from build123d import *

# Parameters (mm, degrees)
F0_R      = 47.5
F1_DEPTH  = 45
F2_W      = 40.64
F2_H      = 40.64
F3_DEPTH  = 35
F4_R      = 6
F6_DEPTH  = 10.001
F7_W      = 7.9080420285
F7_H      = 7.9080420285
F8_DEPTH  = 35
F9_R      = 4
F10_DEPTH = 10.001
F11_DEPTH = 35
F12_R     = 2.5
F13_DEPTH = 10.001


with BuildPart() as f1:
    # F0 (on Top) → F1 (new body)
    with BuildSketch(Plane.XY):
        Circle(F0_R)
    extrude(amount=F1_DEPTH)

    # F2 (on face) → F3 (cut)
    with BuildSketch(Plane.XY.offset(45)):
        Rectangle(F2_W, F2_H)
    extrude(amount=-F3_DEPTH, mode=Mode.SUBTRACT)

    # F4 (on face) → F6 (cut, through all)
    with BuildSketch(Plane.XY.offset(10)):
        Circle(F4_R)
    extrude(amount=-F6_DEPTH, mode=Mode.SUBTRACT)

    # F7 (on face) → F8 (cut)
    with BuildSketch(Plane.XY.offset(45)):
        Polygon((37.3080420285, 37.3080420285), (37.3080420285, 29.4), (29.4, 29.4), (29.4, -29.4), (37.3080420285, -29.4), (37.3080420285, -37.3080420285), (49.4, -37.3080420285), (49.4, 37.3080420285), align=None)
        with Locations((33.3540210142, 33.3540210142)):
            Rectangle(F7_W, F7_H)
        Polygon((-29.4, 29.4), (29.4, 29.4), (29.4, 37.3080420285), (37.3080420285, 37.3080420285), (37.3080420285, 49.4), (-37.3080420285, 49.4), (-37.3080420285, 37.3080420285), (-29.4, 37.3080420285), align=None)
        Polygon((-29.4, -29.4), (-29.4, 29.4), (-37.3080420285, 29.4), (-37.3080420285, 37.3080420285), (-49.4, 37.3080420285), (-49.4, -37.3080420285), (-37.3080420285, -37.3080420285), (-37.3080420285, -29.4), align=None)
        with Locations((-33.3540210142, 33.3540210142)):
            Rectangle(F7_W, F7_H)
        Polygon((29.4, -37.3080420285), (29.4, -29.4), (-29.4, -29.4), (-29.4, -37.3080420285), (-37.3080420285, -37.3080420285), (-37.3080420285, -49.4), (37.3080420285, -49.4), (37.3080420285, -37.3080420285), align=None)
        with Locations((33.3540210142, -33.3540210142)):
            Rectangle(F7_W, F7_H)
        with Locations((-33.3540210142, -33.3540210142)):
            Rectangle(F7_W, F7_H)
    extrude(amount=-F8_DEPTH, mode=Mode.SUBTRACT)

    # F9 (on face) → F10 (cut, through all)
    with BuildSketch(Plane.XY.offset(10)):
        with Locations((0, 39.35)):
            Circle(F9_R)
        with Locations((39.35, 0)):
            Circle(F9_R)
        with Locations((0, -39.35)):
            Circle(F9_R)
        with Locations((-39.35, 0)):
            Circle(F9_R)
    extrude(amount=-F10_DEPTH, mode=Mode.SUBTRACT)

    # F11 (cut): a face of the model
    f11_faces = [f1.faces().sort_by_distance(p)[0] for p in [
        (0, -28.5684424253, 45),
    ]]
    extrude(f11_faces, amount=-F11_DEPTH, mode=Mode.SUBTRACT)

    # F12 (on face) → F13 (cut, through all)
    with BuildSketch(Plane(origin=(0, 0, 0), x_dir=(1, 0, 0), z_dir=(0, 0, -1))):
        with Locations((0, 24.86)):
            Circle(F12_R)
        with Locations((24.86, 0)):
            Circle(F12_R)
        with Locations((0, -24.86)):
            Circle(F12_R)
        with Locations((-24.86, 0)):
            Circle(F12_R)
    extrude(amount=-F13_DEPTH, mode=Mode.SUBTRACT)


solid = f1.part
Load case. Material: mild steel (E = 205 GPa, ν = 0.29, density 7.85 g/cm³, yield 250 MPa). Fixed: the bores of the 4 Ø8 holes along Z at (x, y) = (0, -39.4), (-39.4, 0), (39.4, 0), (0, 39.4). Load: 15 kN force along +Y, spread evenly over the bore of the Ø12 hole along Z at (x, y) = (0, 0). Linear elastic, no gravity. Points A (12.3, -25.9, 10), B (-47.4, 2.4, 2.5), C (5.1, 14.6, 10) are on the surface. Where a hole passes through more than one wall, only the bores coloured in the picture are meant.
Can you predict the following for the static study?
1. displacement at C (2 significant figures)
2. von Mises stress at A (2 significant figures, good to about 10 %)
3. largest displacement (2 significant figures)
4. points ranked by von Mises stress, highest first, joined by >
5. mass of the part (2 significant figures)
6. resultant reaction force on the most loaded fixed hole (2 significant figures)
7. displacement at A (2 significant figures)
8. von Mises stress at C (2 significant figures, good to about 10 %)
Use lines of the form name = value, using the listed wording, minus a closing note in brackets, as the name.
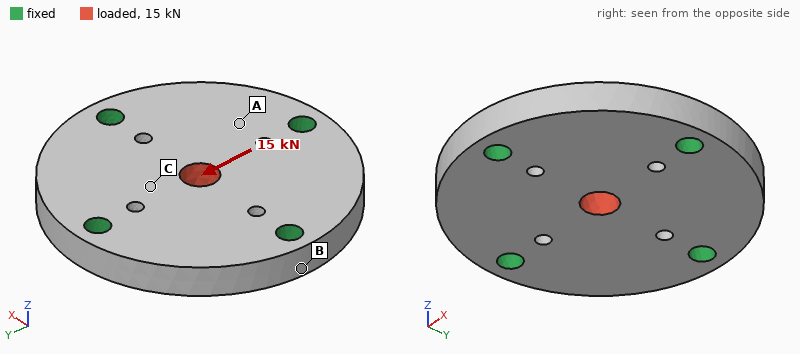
displacement at C = 3.2 µm
von Mises stress at A = 12 MPa
largest displacement = 4.9 µm
points ranked by von Mises stress, highest first, joined by > = C > A > B
mass of the part = 530 g
resultant reaction force on the most loaded fixed hole = 4.8 kN
displacement at A = 2.0 µm
von Mises stress at C = 30 MPa
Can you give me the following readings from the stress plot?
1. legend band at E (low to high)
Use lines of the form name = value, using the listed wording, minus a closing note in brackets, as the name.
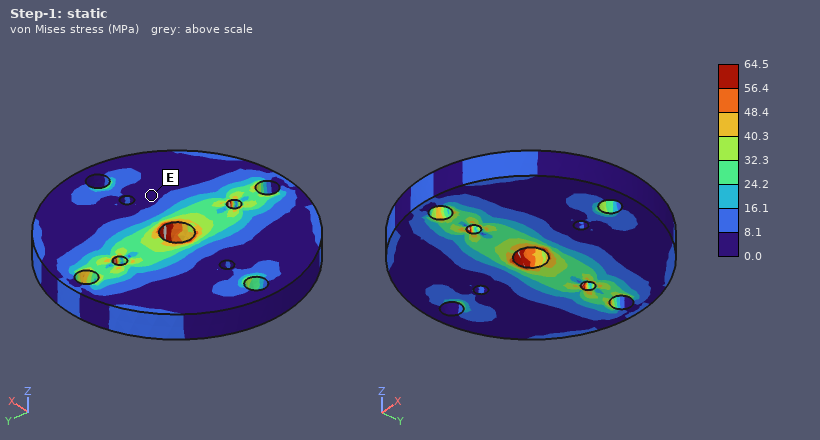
legend band at E = 0.0 to 8.1 MPa
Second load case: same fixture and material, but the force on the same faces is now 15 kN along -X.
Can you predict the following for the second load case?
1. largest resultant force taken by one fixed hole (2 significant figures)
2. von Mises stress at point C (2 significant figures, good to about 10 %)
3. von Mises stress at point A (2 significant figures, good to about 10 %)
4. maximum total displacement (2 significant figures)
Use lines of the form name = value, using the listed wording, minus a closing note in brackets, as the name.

largest resultant force taken by one fixed hole = 4.8 kN
von Mises stress at point C = 11 MPa
von Mises stress at point A = 6.7 MPa
maximum total displacement = 4.9 µm
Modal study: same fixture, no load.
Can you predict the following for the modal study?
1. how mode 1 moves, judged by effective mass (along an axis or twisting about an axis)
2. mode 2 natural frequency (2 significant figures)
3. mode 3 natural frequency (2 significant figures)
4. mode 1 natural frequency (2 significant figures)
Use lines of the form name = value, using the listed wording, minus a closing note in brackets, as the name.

how mode 1 moves, judged by effective mass = along Z
mode 2 natural frequency = 13 kHz
mode 3 natural frequency = 13 kHz
mode 1 natural frequency = 11 kHz
